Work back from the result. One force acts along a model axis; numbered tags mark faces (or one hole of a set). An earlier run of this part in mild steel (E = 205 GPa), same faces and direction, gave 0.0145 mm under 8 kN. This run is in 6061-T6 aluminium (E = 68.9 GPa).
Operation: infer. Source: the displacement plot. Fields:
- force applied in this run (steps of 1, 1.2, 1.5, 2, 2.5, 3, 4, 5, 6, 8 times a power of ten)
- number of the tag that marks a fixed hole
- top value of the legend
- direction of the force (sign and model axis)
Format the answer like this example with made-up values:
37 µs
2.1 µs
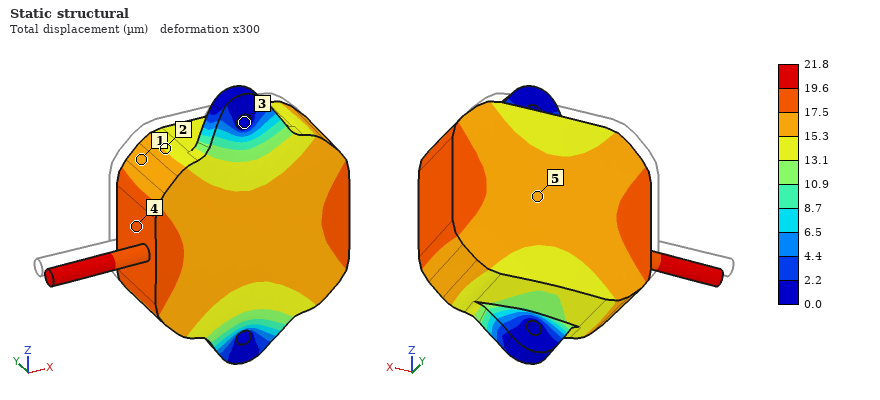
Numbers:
4 kN
3
21.8 µm
-Y
